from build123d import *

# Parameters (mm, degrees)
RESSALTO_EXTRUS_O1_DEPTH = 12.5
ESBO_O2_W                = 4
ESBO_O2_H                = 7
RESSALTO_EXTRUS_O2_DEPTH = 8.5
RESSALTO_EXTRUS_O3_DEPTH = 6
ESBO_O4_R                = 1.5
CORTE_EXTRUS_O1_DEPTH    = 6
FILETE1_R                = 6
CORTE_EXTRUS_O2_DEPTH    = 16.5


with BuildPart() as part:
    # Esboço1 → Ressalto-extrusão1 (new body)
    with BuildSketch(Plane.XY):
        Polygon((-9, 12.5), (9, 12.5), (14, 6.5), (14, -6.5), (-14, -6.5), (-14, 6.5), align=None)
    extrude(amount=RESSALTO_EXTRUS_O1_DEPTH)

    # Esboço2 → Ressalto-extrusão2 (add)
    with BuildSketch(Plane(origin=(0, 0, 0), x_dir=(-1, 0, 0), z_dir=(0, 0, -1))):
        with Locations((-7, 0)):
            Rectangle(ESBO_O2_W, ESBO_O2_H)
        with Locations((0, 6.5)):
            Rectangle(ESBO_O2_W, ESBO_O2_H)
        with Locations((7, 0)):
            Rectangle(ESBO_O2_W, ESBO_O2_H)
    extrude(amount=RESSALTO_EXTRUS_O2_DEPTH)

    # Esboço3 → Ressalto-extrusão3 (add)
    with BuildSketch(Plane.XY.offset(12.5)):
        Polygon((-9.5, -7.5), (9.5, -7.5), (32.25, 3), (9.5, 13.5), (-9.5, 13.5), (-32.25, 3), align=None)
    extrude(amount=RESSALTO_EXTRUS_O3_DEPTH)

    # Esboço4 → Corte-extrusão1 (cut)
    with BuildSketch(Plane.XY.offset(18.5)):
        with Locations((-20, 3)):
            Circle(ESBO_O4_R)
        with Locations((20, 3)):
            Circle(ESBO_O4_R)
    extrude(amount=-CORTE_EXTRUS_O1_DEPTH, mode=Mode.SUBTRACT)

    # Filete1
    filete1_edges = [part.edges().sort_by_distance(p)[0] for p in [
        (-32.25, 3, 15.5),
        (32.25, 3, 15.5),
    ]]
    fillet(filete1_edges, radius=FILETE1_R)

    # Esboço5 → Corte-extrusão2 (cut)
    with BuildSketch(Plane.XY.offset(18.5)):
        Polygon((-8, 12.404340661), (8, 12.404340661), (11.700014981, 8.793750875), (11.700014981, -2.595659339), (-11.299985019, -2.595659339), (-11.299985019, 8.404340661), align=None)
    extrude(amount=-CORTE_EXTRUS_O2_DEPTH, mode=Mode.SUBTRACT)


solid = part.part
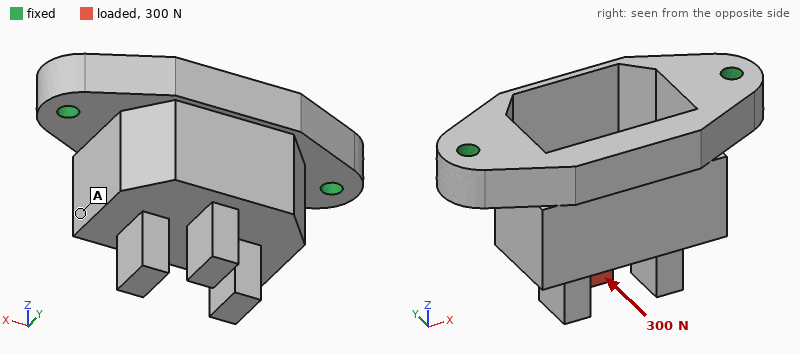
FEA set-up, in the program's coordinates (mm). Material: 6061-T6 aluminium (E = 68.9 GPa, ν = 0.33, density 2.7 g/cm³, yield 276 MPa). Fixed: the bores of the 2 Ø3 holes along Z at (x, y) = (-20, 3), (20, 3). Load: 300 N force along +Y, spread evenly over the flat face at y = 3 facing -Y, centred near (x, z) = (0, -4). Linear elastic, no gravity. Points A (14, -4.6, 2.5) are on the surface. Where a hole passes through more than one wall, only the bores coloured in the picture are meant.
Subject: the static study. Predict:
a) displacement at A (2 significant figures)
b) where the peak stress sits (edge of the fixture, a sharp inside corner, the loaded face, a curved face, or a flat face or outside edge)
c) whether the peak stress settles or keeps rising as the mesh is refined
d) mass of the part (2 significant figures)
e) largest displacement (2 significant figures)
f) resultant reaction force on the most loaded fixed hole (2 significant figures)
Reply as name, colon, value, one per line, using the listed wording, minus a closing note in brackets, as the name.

displacement at A: 22 µm
where the peak stress sits: edge of the fixture
whether the peak stress settles or keeps rising as the mesh is refined: keeps rising
mass of the part: 17 g
largest displacement: 61 µm
resultant reaction force on the most loaded fixed hole: 160 N
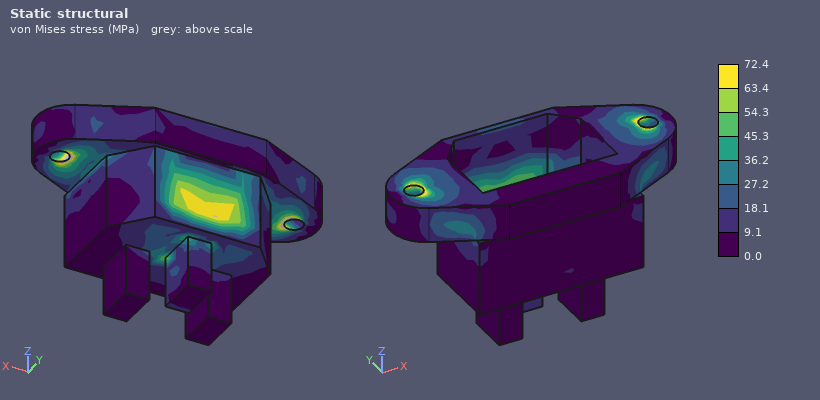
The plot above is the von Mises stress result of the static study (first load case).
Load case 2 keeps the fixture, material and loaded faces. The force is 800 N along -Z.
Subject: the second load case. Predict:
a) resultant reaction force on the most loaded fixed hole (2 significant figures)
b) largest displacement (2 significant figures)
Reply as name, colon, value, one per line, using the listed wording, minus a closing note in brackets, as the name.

resultant reaction force on the most loaded fixed hole: 420 N
largest displacement: 54 µm
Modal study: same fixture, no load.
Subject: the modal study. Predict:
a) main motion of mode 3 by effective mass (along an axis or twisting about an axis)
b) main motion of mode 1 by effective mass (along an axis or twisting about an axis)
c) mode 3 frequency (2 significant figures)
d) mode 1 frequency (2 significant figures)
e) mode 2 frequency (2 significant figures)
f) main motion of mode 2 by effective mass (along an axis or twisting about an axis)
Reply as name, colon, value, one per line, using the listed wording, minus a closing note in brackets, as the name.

main motion of mode 3 by effective mass: along Z
main motion of mode 1 by effective mass: along Y
mode 3 frequency: 15 kHz
mode 1 frequency: 6600 Hz
mode 2 frequency: 13 kHz
main motion of mode 2 by effective mass: along X
